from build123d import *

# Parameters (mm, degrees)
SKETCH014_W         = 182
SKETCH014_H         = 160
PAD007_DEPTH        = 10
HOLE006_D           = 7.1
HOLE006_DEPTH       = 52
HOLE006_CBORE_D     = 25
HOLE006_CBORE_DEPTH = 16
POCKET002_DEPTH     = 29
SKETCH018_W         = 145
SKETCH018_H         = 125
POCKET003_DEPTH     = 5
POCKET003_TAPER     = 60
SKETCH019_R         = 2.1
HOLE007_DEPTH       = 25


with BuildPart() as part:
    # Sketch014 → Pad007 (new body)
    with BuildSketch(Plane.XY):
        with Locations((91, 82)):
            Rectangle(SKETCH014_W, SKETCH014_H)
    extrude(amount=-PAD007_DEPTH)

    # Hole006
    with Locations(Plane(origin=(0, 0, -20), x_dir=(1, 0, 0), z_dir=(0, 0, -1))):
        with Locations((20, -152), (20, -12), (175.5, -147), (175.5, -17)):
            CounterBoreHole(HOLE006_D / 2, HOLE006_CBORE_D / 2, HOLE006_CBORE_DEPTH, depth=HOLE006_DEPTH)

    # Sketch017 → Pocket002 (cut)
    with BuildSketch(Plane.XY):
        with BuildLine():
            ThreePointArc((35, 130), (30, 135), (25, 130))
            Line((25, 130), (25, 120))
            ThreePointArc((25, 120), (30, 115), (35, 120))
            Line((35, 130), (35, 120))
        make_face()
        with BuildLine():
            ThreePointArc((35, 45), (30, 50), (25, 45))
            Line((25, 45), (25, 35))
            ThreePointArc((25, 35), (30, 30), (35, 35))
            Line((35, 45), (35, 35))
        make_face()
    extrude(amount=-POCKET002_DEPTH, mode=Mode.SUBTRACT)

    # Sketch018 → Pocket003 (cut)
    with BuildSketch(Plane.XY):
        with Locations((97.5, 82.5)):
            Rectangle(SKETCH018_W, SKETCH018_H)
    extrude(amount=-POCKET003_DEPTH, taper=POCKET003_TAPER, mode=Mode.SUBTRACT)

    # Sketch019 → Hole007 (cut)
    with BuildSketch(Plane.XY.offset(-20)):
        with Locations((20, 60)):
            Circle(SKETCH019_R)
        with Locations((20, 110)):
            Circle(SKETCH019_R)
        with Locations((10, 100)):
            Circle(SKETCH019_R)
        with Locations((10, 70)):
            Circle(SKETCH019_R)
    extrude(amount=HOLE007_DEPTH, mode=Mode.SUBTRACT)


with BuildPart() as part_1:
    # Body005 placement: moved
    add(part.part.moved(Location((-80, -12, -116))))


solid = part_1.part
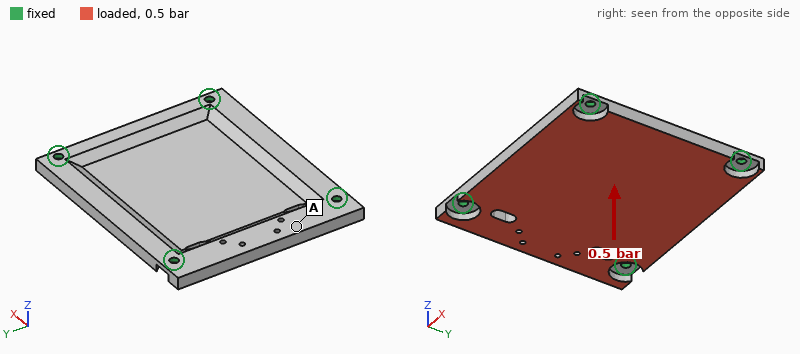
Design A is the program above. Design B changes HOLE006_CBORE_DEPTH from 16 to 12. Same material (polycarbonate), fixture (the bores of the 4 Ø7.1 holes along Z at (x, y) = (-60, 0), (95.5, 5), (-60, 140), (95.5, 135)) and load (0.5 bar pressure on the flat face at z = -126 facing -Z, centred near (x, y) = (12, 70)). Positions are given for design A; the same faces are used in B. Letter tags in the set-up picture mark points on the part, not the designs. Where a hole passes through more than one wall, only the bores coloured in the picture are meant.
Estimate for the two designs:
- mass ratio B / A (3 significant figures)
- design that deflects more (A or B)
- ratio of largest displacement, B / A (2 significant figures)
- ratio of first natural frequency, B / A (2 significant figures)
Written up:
1.03
A
0.82
1.1
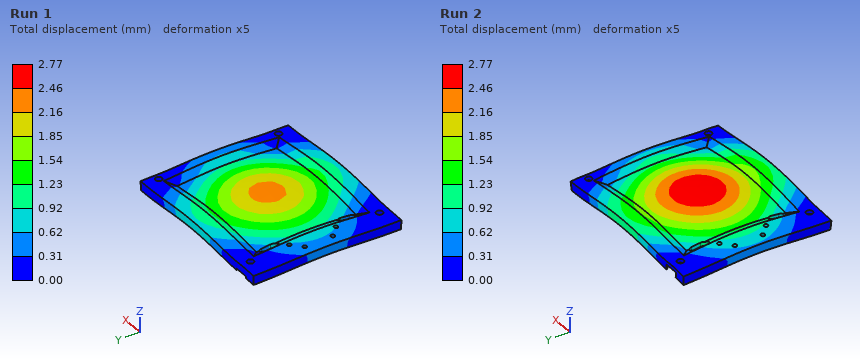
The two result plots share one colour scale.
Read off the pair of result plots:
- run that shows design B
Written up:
Run 1
